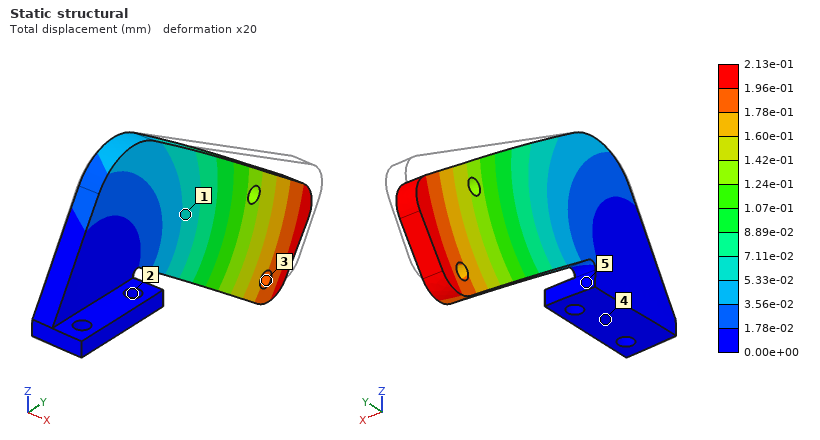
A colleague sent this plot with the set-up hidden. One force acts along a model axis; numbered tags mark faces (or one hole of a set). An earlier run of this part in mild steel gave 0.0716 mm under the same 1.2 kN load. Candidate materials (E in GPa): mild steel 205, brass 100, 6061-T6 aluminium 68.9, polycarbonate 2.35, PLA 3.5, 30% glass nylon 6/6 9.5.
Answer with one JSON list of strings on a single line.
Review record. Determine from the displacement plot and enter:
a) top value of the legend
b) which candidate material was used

["2.13e-01 mm", "6061-T6 aluminium"]
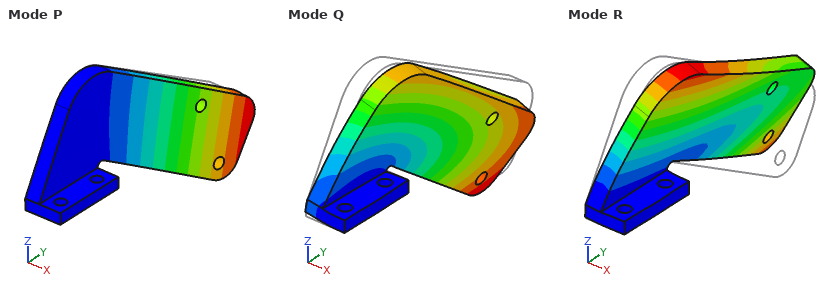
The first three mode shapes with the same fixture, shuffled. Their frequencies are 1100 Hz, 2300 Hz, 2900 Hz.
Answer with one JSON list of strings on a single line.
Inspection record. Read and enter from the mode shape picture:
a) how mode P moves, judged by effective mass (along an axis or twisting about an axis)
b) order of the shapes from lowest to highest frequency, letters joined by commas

["along X", "P, R, Q"]
